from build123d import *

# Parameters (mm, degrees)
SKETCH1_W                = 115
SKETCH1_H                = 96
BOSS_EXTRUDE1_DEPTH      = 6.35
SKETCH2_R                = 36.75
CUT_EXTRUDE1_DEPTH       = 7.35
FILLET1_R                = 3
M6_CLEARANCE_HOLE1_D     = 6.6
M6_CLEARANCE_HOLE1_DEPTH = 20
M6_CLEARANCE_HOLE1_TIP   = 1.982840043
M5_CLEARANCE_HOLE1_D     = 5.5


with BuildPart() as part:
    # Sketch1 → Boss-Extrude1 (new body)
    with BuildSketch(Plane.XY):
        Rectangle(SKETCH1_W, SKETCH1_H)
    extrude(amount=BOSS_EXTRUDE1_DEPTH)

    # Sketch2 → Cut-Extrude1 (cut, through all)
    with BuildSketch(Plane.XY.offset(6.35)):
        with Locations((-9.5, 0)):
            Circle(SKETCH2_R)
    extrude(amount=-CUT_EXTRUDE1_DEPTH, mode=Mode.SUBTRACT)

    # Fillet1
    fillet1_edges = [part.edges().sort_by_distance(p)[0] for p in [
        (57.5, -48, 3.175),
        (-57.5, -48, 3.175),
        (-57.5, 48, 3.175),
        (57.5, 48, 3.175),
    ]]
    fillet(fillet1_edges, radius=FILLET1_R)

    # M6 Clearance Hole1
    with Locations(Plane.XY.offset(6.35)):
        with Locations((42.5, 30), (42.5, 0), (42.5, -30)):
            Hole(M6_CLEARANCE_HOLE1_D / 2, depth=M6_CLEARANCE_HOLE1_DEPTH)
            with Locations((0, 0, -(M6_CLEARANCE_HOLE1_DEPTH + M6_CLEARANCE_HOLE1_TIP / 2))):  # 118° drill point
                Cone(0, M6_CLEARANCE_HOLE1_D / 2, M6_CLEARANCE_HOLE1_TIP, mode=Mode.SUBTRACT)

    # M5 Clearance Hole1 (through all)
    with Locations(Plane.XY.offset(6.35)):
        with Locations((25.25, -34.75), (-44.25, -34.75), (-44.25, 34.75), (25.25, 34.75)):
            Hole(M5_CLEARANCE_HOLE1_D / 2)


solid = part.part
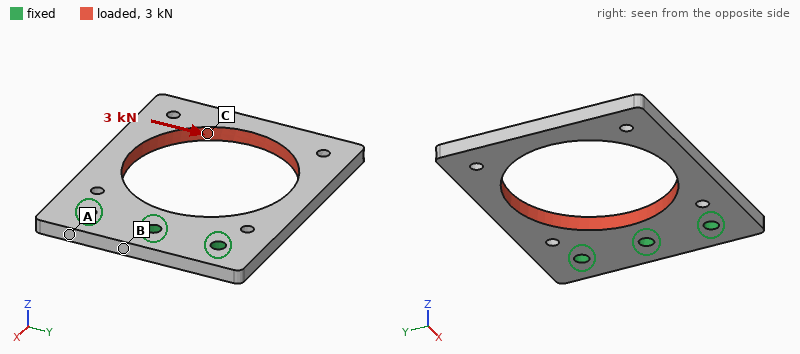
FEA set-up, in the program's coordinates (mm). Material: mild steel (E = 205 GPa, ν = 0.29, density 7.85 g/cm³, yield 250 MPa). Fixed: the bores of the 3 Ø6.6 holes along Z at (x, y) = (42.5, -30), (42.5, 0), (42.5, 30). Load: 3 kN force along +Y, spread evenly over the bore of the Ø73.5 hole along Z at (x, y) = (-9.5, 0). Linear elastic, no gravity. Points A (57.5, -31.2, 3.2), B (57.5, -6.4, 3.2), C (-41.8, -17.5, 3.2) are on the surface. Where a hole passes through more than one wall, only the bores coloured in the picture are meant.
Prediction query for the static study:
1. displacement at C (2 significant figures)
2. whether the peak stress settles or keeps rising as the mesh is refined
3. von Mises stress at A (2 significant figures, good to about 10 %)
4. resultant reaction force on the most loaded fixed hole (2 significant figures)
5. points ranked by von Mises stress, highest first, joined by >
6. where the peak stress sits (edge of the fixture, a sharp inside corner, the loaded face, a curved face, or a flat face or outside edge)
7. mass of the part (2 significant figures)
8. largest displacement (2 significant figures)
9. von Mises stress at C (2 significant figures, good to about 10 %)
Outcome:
67 µm
keeps rising
21 MPa
2.3 kN
C > A > B
edge of the fixture
330 g
73 µm
43 MPa
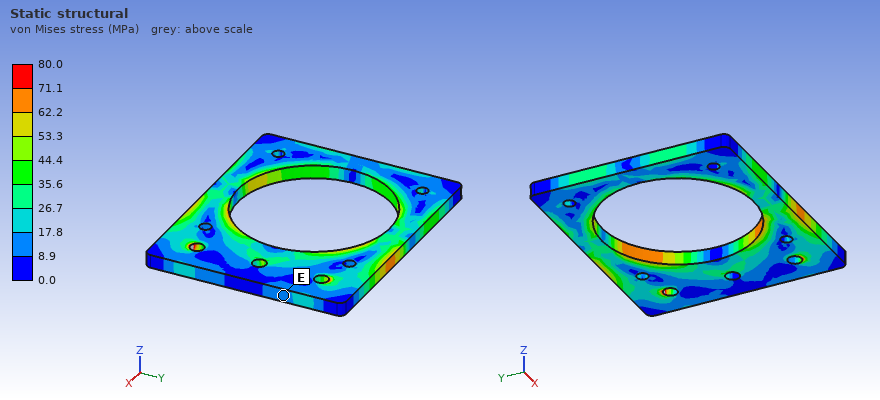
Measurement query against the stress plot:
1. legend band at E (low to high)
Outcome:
8.9 to 17.8 MPa
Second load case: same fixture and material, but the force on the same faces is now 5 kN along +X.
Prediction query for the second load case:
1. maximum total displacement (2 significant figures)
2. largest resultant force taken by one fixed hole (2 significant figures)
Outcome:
26 µm
2.7 kN
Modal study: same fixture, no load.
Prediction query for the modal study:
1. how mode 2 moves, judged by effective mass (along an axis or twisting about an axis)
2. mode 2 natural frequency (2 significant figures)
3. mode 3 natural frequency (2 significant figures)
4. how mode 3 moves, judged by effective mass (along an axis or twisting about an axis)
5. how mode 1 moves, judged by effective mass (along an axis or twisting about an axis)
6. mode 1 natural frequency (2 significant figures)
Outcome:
twisting about X
980 Hz
2200 Hz
along Y
along Z
420 Hz
